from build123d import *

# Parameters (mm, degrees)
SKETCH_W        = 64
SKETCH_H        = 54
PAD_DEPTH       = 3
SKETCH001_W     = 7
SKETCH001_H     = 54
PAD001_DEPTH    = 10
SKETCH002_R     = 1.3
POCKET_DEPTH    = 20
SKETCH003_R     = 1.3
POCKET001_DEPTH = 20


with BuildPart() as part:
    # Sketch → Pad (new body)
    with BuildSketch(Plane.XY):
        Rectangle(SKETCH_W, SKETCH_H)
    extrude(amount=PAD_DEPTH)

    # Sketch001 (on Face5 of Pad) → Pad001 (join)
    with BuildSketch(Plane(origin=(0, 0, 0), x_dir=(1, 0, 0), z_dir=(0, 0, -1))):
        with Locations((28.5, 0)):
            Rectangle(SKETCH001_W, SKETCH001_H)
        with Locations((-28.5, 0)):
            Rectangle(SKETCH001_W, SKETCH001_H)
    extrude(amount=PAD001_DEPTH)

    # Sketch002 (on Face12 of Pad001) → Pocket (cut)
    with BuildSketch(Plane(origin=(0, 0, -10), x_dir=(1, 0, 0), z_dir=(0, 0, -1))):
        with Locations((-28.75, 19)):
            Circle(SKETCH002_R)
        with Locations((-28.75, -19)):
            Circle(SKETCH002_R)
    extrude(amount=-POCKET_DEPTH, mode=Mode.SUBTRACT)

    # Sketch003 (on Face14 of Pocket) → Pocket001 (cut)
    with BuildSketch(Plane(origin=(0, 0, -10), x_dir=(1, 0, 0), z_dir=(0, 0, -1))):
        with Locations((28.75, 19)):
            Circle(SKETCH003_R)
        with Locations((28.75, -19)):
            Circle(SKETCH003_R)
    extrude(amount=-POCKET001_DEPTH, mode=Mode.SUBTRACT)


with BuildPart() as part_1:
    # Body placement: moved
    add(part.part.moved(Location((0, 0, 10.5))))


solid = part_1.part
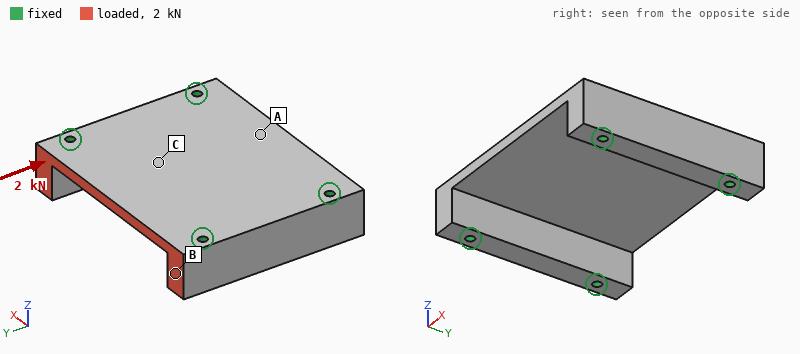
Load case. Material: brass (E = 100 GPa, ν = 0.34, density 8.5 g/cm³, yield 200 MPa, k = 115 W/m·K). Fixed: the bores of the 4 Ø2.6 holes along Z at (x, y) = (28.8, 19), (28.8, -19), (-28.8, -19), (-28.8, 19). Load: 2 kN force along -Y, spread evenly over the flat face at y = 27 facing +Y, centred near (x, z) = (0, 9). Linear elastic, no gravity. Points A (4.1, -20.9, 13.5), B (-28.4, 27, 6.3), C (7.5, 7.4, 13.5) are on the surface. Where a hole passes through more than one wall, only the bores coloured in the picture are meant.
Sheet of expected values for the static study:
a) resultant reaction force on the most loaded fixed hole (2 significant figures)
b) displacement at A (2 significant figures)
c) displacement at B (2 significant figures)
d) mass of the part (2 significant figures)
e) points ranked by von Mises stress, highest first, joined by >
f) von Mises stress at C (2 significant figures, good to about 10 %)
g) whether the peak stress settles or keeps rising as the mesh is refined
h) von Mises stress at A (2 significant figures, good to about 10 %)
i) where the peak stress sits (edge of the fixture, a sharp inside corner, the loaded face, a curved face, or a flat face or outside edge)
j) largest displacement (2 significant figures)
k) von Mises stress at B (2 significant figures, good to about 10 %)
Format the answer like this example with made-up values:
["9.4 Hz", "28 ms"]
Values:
["800 N", "1.1 µm", "0.65 µm", "150 g", "B > C > A", "4.6 MPa", "keeps rising", "1.6 MPa", "edge of the fixture", "2.7 µm", "6.9 MPa"]
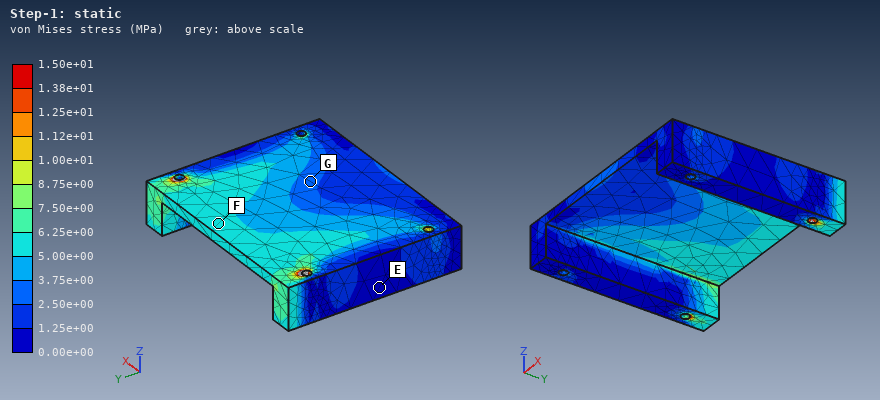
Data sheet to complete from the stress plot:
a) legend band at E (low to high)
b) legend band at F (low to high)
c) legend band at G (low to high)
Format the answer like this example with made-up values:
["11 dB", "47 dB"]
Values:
["0.00e+00 to 1.25e+00 MPa", "5.00e+00 to 6.25e+00 MPa", "2.50e+00 to 3.75e+00 MPa"]
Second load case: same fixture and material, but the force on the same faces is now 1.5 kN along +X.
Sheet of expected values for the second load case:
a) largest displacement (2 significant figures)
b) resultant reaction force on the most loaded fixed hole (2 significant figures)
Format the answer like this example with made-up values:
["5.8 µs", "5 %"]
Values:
["3.7 µm", "720 N"]
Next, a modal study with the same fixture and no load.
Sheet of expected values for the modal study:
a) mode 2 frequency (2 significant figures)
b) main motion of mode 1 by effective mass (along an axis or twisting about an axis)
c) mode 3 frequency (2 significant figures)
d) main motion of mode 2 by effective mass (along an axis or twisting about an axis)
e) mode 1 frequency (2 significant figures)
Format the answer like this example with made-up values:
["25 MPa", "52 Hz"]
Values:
["4400 Hz", "along Z", "7000 Hz", "twisting about X", "3700 Hz"]
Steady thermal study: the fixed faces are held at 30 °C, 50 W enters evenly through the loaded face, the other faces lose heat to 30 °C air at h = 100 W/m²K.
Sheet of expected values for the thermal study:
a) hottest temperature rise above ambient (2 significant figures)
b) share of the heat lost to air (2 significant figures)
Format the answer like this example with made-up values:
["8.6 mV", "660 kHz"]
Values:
["27 K", "9.2 %"]
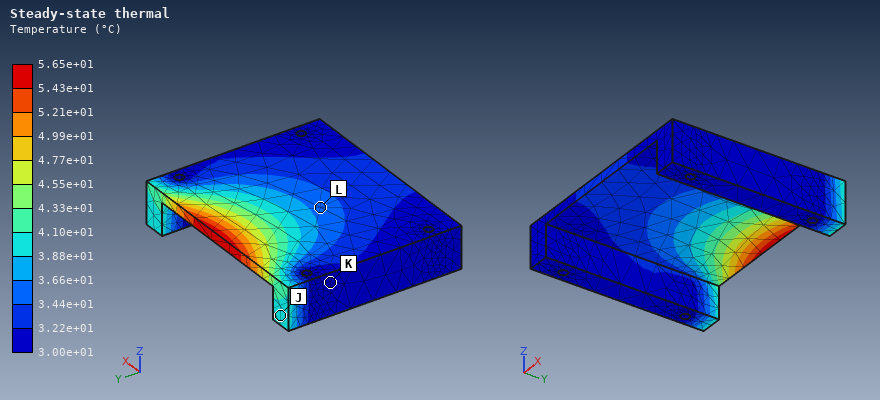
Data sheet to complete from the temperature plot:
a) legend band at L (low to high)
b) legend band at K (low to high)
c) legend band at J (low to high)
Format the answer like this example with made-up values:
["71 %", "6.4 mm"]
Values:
["3.44e+01 to 3.66e+01 °C", "3.00e+01 to 3.22e+01 °C", "3.88e+01 to 4.10e+01 °C"]
